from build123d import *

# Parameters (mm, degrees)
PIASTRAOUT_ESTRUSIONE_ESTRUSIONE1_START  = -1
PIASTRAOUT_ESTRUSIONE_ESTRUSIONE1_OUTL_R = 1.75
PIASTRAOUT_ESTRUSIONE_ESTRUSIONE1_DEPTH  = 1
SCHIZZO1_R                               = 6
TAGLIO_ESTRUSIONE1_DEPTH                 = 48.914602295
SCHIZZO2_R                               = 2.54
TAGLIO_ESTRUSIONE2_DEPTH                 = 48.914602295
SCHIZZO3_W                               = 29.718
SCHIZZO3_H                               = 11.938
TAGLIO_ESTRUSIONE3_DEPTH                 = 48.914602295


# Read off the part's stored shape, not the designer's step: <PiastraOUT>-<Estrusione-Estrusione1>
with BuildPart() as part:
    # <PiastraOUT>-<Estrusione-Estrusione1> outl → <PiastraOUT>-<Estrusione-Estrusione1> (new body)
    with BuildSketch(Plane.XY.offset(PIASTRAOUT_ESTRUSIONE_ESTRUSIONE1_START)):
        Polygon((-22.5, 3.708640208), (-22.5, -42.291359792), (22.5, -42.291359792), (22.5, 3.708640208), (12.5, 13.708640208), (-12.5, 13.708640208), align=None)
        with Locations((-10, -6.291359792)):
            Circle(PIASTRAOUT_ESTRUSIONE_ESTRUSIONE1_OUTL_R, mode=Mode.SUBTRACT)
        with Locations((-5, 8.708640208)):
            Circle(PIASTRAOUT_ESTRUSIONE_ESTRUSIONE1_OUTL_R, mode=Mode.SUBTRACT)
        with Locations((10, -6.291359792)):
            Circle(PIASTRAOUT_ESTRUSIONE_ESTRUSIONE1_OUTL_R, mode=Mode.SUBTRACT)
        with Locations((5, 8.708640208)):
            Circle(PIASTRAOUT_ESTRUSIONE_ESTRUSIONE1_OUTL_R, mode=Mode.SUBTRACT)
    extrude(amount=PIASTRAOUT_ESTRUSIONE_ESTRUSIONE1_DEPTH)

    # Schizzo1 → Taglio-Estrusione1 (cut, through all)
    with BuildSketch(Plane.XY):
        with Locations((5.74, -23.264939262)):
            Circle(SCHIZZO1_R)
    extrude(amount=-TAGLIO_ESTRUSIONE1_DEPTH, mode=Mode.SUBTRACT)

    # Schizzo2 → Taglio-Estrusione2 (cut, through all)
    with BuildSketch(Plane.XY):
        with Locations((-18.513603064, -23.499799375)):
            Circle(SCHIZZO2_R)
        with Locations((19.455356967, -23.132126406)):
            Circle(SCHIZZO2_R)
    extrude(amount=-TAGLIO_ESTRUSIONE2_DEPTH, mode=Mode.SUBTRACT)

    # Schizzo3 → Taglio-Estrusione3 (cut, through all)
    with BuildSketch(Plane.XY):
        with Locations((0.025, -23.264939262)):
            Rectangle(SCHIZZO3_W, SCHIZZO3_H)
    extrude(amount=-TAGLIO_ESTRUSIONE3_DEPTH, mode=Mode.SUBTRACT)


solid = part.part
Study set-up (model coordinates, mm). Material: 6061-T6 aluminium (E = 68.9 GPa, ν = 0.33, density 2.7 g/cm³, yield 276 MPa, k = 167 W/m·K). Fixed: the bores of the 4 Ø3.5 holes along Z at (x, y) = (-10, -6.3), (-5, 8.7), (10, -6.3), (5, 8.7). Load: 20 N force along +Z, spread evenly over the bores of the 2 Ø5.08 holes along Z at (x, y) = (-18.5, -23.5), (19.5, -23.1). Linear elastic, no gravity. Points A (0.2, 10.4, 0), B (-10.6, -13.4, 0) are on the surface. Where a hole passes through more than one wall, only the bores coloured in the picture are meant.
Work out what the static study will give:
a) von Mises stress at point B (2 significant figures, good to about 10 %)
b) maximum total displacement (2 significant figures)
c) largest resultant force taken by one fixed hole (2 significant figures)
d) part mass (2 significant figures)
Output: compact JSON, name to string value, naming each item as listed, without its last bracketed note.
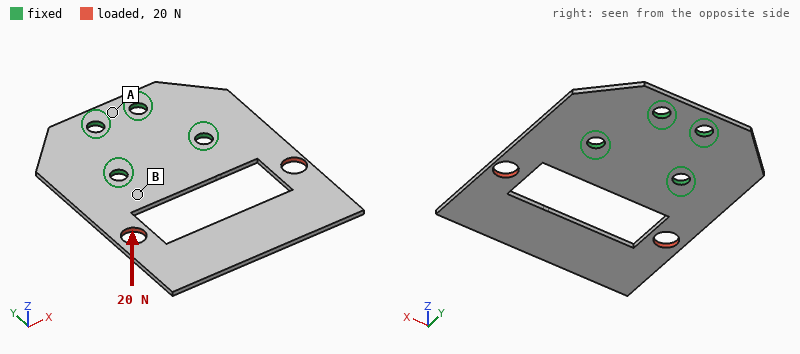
{"von Mises stress at point B": "39 MPa", "maximum total displacement": "0.66 mm", "largest resultant force taken by one fixed hole": "13 N", "part mass": "5.4 g"}
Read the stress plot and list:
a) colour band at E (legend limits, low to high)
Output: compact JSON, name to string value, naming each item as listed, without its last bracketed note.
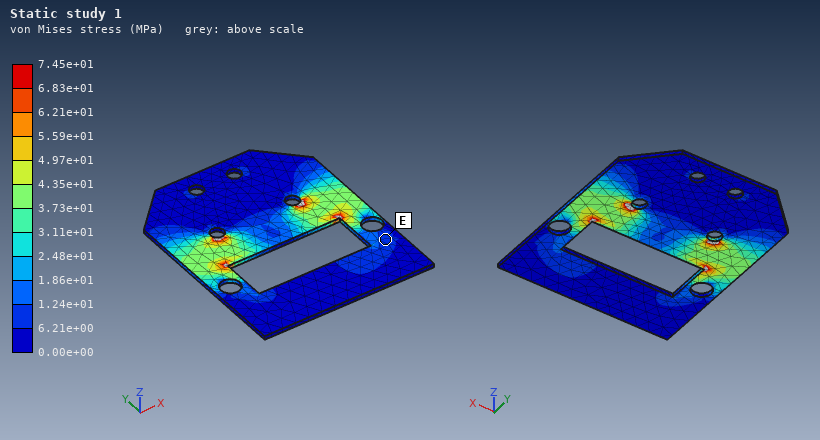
{"colour band at E": "6.21e+00 to 1.24e+01 MPa"}
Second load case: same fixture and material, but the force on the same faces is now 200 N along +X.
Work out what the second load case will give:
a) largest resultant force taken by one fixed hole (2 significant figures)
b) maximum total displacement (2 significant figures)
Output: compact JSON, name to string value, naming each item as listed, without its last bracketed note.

{"largest resultant force taken by one fixed hole": "160 N", "maximum total displacement": "44 µm"}
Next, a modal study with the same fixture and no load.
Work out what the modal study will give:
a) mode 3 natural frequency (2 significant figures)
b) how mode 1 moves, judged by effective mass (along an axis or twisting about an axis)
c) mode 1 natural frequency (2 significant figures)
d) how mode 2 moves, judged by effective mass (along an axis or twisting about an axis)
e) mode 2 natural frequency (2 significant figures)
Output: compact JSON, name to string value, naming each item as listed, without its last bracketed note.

{"mode 3 natural frequency": "2800 Hz", "how mode 1 moves, judged by effective mass": "along Z", "mode 1 natural frequency": "430 Hz", "how mode 2 moves, judged by effective mass": "twisting about Y", "mode 2 natural frequency": "1100 Hz"}
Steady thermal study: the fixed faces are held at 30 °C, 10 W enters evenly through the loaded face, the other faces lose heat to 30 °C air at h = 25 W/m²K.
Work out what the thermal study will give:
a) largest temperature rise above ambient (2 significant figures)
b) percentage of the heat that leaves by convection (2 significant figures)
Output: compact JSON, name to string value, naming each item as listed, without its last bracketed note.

{"largest temperature rise above ambient": "58 K", "percentage of the heat that leaves by convection": "22 %"}
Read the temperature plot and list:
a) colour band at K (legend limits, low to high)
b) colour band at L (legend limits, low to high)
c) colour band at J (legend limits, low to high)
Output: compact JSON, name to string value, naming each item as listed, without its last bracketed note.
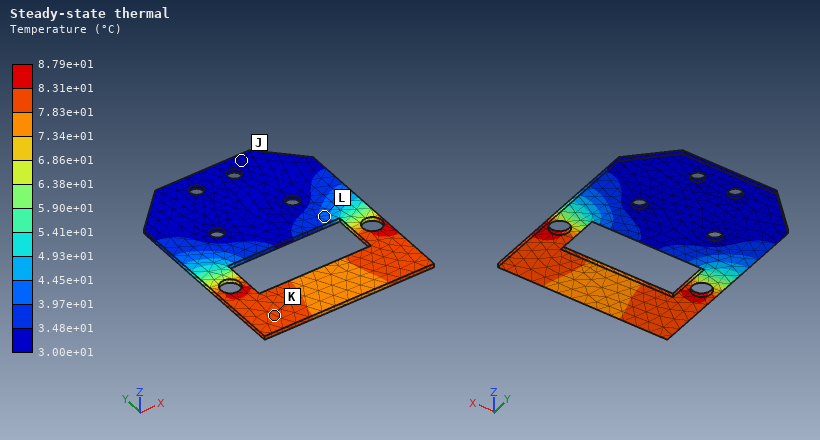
{"colour band at K": "7.83e+01 to 8.31e+01 °C", "colour band at L": "3.97e+01 to 4.45e+01 °C", "colour band at J": "3.00e+01 to 3.48e+01 °C"}
